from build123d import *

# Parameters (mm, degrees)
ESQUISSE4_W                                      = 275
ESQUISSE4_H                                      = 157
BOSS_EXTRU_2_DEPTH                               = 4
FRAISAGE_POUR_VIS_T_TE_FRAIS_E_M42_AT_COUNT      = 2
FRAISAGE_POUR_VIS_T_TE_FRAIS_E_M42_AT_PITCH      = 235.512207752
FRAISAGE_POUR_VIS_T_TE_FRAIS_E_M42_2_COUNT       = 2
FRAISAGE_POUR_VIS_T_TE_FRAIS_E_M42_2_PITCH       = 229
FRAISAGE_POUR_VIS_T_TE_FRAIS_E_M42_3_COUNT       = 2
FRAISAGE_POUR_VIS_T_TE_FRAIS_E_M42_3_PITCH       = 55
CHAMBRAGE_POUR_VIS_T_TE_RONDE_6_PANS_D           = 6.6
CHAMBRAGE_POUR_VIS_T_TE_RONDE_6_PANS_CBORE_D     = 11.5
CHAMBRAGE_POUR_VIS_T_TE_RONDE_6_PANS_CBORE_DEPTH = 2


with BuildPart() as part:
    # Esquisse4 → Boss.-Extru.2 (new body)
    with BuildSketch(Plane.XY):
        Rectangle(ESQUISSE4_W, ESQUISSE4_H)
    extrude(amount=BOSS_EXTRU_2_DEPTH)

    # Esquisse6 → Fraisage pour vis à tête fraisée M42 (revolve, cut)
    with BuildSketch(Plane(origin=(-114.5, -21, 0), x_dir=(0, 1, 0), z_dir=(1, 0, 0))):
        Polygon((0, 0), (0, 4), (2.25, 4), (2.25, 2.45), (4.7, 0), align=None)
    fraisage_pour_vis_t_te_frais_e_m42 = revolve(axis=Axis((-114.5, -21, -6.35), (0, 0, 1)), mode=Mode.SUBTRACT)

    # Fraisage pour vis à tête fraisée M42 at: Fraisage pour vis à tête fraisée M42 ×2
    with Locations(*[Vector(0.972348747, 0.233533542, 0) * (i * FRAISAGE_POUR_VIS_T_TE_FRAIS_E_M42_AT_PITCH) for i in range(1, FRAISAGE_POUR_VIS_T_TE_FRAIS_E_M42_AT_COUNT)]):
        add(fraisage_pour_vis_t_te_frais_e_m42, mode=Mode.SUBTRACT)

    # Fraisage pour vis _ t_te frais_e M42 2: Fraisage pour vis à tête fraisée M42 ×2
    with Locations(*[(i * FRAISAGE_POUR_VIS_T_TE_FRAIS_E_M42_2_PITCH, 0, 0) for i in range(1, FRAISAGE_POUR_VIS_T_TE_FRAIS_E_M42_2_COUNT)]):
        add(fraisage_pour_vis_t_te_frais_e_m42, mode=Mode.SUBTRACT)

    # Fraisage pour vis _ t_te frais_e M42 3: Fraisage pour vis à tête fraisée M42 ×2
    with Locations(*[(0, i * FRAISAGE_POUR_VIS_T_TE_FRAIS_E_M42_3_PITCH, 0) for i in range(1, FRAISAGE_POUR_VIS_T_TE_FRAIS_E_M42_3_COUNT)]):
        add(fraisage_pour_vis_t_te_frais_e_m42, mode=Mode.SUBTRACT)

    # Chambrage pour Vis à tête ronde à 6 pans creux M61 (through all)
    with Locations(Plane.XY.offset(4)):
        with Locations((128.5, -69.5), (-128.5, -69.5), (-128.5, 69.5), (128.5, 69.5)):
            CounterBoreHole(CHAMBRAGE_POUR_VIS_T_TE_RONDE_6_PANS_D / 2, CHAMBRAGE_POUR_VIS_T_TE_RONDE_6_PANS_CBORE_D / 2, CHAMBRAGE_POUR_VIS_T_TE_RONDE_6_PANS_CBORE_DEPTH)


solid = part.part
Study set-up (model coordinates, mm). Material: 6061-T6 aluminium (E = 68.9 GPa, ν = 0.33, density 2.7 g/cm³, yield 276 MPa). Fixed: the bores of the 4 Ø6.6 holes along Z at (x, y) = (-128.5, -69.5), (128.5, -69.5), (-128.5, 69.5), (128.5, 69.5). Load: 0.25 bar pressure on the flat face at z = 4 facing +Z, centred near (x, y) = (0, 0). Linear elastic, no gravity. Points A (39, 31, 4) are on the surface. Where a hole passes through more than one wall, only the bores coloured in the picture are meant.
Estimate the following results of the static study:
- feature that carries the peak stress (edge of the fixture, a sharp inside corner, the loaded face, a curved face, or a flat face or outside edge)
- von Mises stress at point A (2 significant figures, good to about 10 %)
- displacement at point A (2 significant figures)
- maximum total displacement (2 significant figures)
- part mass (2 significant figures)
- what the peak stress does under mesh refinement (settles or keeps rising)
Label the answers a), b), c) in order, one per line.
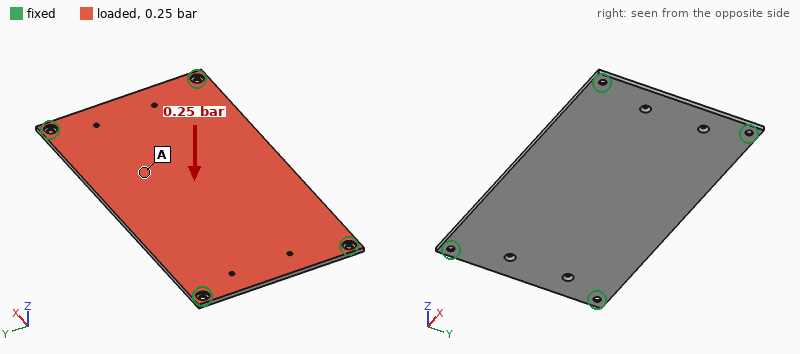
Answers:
a) edge of the fixture
b) 29 MPa
c) 1.2 mm
d) 1.4 mm
e) 460 g
f) keeps rising
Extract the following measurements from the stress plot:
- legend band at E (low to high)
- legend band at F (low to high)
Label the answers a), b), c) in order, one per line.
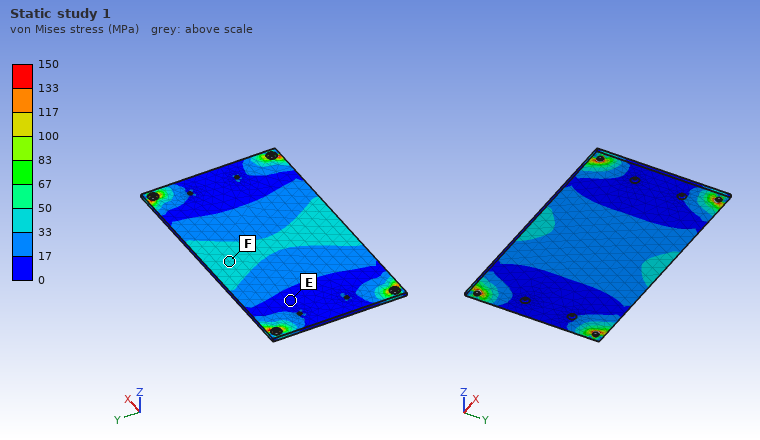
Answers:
a) 0 to 17 MPa
b) 33 to 50 MPa
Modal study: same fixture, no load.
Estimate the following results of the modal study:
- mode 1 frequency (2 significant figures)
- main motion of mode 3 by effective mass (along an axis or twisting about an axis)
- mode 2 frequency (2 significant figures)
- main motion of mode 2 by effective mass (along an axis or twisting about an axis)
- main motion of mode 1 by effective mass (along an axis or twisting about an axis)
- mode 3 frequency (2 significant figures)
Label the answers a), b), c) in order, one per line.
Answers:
a) 230 Hz
b) twisting about Y
c) 430 Hz
d) twisting about X
e) along Z
f) 640 Hz
